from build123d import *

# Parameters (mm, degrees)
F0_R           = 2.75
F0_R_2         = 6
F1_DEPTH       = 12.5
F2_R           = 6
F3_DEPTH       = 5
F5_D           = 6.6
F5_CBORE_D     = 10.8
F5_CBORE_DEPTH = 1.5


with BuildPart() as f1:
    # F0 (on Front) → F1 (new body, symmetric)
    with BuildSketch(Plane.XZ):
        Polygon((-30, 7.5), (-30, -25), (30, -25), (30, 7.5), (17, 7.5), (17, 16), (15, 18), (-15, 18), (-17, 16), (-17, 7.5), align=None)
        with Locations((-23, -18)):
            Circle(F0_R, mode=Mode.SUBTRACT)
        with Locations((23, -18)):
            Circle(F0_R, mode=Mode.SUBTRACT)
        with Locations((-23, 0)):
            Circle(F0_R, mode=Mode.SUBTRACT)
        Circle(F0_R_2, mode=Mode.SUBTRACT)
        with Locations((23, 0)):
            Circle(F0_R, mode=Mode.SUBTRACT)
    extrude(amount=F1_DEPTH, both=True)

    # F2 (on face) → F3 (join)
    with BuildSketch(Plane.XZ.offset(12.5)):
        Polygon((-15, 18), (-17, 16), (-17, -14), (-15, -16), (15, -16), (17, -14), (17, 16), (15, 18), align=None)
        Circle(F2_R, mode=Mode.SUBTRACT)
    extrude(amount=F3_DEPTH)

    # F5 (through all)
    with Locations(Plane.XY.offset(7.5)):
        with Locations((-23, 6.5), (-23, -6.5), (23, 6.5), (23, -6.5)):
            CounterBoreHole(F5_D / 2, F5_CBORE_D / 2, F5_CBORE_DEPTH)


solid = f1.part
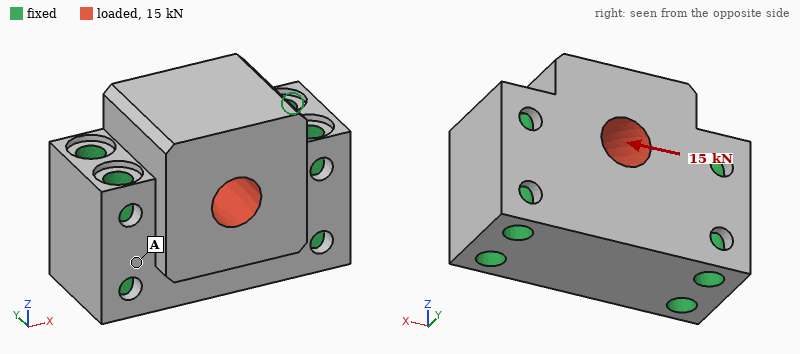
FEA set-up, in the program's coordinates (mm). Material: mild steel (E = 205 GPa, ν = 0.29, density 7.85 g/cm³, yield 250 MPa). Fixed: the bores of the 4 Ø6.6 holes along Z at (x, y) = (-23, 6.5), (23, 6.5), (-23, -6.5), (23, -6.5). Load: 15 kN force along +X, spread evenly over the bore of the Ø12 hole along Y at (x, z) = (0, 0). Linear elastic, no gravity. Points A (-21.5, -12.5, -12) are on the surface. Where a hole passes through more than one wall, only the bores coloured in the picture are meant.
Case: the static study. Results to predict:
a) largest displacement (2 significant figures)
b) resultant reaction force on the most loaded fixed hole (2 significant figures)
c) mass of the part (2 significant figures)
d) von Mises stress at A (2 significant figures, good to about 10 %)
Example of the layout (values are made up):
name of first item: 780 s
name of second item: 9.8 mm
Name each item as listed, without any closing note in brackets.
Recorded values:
largest displacement: 1.8 µm
resultant reaction force on the most loaded fixed hole: 4.2 kN
mass of the part: 420 g
von Mises stress at A: 6.3 MPa
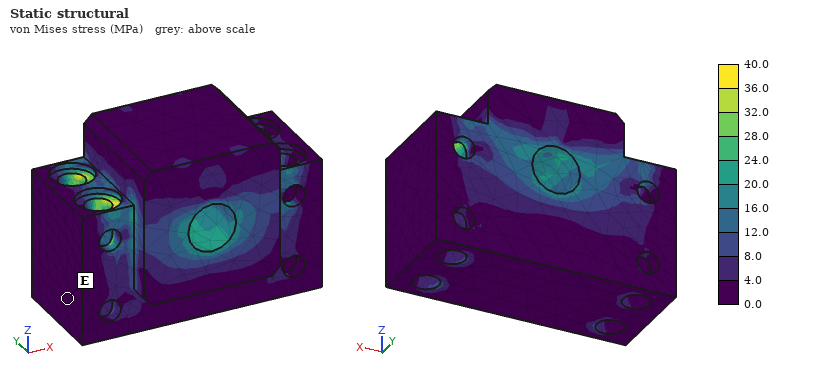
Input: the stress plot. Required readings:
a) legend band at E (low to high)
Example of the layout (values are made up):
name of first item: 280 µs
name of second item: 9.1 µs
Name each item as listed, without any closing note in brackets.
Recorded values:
legend band at E: 0.0 to 4.0 MPa
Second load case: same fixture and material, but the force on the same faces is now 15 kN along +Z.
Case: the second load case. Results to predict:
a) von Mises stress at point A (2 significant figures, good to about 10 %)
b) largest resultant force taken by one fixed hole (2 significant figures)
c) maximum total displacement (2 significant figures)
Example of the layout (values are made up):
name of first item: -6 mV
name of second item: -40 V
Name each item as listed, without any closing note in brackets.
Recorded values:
von Mises stress at point A: 11 MPa
largest resultant force taken by one fixed hole: 4.5 kN
maximum total displacement: 3.2 µm
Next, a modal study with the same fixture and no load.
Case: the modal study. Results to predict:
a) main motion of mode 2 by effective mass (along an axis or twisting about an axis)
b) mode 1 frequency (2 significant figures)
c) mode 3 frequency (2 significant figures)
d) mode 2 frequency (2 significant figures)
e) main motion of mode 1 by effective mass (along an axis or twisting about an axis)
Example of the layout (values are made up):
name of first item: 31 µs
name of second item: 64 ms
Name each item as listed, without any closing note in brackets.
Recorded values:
main motion of mode 2 by effective mass: along Z
mode 1 frequency: 19 kHz
mode 3 frequency: 32 kHz
mode 2 frequency: 30 kHz
main motion of mode 1 by effective mass: along Y
